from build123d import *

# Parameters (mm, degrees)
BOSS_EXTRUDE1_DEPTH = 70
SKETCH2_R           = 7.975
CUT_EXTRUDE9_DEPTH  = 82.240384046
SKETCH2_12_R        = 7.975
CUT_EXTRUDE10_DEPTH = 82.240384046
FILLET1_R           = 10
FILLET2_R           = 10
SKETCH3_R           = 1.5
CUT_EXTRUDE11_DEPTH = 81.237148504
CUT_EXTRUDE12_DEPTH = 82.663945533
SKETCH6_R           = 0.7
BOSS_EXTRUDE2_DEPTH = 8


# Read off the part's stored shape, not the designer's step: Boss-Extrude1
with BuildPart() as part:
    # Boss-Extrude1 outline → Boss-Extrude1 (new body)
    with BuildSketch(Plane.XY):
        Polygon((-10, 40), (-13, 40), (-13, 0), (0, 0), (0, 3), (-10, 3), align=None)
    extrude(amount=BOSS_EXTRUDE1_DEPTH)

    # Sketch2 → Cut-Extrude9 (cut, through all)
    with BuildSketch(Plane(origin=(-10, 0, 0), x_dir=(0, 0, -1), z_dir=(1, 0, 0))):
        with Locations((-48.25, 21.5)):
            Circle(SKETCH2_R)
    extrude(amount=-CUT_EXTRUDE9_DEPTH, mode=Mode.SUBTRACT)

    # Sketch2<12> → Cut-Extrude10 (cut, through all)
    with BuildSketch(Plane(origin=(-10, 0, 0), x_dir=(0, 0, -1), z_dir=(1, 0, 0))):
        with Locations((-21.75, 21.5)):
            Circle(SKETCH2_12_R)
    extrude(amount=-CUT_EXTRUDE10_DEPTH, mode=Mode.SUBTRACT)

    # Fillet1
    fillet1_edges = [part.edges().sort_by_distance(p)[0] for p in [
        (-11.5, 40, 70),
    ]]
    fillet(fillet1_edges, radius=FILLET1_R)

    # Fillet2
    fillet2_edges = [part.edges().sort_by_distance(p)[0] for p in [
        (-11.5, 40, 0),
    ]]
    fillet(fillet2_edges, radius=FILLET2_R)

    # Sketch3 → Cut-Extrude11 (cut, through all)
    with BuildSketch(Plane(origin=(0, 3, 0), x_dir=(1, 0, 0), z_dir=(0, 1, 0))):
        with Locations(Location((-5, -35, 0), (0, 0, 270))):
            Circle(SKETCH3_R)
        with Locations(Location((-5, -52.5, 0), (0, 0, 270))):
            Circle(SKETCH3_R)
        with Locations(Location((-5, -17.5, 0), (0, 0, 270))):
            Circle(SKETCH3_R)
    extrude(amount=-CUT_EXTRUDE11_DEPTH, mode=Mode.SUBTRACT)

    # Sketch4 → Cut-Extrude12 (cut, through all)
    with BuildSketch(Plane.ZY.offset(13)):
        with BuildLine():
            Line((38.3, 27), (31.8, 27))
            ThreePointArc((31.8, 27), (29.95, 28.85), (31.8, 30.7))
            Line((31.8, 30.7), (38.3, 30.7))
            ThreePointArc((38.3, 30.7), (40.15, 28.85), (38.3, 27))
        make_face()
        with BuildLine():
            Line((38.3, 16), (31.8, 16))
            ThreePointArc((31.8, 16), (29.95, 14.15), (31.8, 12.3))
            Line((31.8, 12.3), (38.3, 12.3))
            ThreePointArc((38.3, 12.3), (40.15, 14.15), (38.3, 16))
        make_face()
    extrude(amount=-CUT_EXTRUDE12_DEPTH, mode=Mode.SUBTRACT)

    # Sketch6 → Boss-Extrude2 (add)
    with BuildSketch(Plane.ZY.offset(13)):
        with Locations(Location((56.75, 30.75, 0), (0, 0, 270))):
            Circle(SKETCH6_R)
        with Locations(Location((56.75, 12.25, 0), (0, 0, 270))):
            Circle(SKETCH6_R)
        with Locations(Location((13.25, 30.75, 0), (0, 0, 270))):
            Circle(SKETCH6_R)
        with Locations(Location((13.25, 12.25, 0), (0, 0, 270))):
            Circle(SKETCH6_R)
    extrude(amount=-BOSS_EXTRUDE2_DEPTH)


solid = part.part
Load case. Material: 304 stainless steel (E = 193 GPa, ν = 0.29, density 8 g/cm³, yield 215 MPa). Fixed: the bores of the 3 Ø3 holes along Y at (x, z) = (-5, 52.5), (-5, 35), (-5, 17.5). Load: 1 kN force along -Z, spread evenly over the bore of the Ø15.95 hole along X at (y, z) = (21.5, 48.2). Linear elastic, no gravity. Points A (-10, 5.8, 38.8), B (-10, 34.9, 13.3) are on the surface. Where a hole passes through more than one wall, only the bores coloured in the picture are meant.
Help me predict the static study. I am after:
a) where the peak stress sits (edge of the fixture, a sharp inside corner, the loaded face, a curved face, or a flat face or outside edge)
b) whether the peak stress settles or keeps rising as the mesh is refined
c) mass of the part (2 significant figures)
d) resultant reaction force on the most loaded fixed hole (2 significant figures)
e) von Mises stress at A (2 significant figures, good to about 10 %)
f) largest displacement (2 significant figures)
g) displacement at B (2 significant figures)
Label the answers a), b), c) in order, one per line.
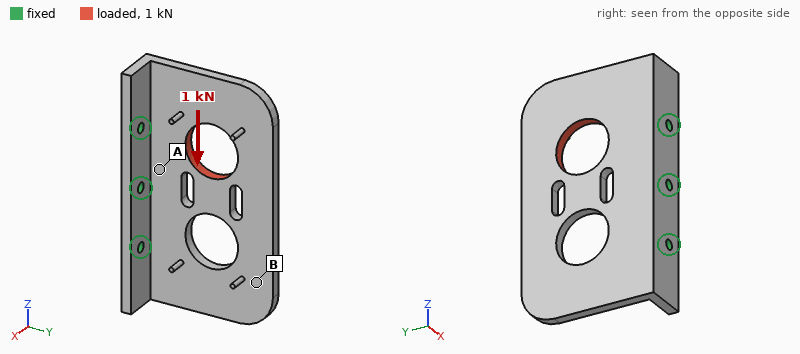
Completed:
a) edge of the fixture
b) keeps rising
c) 71 g
d) 650 N
e) 34 MPa
f) 33 µm
g) 25 µm
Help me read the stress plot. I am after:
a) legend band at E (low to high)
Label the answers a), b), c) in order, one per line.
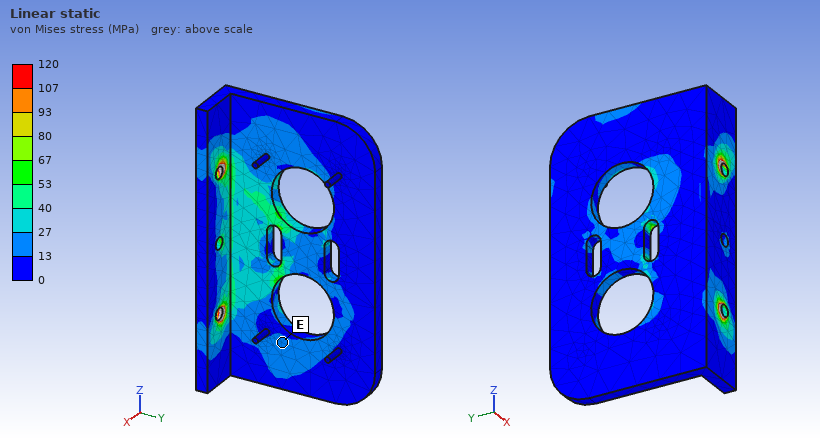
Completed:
a) 13 to 27 MPa
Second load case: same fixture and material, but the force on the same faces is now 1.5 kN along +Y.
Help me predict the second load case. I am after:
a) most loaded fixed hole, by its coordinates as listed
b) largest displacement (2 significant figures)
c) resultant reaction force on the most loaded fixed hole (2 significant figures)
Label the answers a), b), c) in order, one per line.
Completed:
a) (-5, 52.5)
b) 82 µm
c) 1.1 kN
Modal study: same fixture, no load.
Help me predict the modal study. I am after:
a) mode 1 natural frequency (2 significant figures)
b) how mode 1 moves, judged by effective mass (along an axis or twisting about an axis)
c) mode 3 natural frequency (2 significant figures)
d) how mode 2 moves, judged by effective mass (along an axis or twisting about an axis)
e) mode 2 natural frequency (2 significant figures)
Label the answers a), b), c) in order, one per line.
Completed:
a) 1200 Hz
b) along X
c) 4600 Hz
d) twisting about Y
e) 2100 Hz
